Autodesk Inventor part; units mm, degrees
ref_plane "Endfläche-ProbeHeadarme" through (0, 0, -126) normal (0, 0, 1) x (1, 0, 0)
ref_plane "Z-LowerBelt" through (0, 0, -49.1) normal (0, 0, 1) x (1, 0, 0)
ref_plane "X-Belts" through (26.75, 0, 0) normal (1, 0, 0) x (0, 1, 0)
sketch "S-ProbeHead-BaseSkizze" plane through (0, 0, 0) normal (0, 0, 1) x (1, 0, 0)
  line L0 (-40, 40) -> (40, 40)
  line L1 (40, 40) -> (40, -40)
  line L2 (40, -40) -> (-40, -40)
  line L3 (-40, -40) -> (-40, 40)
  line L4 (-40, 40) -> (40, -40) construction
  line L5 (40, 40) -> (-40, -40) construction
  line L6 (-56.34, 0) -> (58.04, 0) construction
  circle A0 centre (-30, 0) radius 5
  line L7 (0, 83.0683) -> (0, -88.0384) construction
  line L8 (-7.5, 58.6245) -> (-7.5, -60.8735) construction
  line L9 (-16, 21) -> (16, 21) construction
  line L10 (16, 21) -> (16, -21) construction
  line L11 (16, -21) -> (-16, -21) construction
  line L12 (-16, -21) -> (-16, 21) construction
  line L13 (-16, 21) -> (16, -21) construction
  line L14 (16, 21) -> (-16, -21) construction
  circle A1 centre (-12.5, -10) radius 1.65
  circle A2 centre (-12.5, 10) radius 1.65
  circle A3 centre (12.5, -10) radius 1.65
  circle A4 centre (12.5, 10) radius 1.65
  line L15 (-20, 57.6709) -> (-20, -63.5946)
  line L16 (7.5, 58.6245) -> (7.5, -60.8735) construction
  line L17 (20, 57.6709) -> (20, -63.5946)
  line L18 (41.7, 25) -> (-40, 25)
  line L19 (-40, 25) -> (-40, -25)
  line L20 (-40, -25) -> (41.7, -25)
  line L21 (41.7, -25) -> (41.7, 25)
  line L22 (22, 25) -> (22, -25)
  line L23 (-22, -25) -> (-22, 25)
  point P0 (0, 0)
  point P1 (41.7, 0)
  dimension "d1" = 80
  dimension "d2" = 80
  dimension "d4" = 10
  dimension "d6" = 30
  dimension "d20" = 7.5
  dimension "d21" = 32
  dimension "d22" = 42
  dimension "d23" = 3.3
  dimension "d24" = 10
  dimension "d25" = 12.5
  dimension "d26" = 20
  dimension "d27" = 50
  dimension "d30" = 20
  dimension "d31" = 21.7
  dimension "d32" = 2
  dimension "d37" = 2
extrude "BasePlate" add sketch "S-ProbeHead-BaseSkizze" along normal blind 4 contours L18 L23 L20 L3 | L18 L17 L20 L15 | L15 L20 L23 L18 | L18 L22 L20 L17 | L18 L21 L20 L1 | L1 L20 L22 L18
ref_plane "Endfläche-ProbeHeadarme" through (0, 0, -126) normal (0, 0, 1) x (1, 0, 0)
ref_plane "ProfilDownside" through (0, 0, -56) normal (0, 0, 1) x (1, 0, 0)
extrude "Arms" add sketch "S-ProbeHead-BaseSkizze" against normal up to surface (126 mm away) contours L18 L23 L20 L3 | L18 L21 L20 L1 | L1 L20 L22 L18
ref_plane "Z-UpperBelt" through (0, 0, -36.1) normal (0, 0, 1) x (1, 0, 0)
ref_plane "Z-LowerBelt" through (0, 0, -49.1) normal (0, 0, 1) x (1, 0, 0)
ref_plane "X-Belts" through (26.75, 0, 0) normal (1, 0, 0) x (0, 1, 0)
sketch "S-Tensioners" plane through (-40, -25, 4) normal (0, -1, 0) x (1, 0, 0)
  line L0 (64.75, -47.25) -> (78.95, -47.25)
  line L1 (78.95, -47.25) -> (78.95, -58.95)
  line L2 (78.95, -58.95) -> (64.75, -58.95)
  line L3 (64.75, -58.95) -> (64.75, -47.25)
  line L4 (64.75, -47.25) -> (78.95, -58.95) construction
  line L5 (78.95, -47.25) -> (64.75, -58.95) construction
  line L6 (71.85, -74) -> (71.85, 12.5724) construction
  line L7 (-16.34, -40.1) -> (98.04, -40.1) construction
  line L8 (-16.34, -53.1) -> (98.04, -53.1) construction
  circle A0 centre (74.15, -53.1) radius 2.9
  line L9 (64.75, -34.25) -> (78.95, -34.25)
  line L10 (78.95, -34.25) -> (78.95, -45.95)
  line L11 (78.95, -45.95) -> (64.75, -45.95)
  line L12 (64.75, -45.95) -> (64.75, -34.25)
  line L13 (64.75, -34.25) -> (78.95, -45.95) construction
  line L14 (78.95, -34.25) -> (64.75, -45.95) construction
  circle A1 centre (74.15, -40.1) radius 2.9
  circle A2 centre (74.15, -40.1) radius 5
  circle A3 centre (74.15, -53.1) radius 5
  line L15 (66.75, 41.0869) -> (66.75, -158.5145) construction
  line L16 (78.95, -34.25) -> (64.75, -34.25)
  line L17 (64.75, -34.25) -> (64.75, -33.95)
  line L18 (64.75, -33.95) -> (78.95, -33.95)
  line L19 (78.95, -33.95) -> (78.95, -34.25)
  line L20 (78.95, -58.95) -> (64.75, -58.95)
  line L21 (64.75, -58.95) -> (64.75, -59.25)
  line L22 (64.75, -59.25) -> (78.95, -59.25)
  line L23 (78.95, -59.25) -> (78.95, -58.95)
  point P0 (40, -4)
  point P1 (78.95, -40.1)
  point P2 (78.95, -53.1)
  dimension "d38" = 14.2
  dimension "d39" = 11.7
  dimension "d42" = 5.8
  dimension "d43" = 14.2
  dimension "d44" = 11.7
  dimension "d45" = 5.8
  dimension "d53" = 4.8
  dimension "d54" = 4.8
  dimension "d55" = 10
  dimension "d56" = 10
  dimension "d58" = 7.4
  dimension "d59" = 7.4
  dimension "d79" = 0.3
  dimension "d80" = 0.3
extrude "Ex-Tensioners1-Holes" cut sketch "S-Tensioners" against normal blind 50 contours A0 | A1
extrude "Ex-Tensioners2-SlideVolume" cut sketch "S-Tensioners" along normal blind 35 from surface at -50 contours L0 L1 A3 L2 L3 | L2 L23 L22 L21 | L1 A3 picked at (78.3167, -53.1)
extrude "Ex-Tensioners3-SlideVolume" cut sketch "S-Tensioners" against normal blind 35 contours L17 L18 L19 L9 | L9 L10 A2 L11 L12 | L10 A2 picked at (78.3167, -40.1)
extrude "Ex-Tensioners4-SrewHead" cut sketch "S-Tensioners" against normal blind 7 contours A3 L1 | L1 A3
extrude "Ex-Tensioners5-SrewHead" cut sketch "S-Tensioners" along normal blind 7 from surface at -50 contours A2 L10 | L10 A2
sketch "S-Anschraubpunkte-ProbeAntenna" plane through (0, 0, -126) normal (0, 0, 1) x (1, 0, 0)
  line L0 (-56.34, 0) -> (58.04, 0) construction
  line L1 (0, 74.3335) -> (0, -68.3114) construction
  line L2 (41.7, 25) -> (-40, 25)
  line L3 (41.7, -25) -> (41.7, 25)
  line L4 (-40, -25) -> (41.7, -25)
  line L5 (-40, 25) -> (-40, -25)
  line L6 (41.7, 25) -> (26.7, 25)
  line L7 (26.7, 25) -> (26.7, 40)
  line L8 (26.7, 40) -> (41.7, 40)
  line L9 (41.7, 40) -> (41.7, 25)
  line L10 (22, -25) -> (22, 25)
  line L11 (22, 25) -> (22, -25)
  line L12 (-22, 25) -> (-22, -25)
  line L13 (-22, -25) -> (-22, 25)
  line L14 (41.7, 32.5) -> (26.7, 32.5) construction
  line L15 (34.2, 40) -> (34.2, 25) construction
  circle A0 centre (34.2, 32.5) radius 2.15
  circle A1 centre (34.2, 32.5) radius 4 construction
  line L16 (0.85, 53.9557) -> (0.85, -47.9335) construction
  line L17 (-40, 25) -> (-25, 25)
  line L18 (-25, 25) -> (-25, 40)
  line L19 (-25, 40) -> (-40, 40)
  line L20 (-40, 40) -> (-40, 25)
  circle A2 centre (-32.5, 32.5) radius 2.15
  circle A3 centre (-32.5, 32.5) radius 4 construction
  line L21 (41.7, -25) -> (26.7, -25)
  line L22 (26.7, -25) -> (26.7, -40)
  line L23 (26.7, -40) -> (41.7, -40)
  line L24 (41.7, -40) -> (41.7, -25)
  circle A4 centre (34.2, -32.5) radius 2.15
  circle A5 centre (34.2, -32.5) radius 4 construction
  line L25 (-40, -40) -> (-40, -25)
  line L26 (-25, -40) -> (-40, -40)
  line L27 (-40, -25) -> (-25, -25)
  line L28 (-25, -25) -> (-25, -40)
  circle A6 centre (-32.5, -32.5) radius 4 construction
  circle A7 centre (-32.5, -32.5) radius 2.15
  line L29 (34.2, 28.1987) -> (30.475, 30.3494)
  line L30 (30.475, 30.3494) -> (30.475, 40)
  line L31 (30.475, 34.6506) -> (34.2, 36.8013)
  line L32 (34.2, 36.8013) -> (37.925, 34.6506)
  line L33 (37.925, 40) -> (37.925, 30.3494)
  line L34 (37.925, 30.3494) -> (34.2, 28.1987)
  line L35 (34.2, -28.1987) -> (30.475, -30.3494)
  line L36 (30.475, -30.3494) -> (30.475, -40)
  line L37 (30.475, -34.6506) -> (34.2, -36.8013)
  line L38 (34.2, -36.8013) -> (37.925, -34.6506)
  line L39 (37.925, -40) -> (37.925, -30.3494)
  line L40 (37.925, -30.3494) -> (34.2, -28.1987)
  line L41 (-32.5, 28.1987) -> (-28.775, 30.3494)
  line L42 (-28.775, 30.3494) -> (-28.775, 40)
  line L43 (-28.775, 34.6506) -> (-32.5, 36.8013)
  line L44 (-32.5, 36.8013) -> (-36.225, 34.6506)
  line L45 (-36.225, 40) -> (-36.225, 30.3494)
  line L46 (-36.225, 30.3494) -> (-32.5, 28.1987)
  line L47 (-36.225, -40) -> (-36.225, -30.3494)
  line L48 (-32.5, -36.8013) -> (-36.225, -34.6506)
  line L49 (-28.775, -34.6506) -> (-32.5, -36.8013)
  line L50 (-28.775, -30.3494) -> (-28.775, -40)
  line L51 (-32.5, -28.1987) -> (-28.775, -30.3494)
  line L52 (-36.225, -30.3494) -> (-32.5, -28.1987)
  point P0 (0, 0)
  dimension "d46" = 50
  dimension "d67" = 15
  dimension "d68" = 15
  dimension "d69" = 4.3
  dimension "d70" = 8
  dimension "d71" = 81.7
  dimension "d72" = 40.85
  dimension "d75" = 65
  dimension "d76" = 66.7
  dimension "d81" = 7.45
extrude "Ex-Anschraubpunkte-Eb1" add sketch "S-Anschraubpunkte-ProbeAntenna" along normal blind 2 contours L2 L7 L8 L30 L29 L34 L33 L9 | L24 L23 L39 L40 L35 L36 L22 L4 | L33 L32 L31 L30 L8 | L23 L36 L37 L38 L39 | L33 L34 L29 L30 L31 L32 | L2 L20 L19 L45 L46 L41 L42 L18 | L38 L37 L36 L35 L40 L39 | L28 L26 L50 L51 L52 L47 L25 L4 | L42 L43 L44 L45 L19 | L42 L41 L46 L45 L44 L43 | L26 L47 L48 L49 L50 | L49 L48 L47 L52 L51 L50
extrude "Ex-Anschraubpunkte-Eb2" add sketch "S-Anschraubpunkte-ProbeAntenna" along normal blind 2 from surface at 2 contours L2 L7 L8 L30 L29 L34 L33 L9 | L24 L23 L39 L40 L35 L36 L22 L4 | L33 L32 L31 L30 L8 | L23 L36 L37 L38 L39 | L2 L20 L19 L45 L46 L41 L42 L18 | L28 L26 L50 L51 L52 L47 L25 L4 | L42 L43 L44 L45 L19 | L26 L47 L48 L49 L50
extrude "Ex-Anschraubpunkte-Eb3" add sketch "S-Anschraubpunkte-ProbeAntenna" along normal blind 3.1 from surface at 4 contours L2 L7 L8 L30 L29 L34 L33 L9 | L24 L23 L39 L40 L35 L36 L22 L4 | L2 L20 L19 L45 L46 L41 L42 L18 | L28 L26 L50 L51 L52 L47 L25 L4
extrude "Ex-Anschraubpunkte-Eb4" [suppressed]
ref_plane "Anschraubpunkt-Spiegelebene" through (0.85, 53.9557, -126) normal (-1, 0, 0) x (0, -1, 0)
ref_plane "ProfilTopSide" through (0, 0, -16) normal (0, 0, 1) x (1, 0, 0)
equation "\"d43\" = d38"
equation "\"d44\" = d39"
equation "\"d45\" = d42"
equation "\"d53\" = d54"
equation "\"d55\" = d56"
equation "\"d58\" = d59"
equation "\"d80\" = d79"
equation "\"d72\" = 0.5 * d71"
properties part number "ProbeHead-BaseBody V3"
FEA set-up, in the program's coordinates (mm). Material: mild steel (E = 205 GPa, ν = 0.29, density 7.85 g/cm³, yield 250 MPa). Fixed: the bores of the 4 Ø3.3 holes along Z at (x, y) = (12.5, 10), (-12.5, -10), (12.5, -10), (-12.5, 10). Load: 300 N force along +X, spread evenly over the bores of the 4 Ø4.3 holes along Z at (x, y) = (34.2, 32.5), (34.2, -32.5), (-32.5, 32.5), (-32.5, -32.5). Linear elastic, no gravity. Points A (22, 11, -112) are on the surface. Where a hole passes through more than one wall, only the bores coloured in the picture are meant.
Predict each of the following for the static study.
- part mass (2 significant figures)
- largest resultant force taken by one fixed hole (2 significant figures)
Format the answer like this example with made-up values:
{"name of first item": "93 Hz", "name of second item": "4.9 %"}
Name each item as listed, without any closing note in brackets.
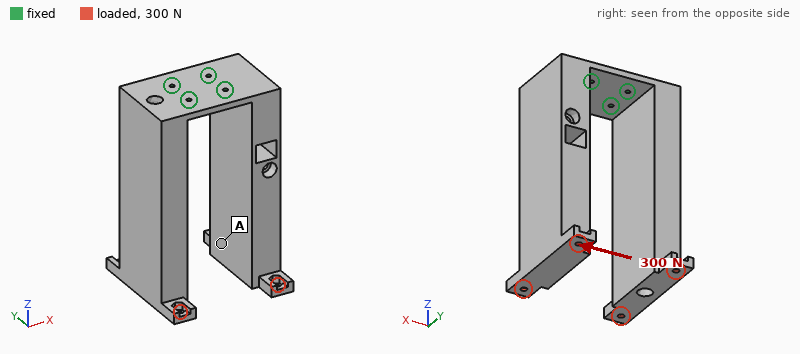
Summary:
{"part mass": "1.8 kg", "largest resultant force taken by one fixed hole": "290 N"}
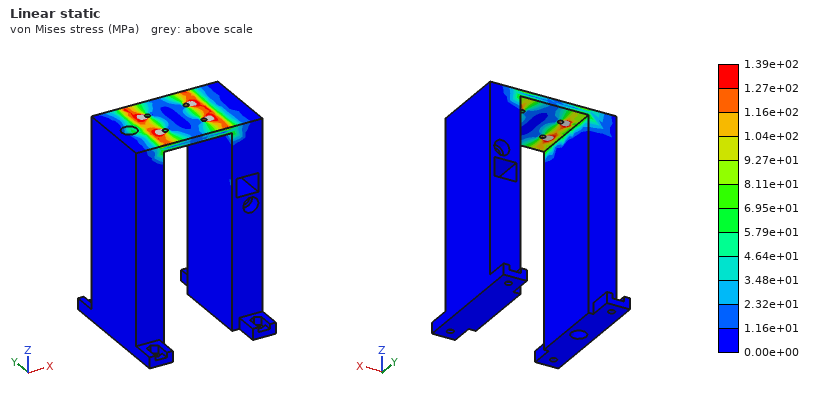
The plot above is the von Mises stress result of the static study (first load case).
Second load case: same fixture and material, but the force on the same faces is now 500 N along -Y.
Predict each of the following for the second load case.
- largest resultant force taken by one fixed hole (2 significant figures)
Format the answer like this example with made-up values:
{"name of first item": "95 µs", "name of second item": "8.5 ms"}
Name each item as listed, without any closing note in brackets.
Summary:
{"largest resultant force taken by one fixed hole": "1.3 kN"}
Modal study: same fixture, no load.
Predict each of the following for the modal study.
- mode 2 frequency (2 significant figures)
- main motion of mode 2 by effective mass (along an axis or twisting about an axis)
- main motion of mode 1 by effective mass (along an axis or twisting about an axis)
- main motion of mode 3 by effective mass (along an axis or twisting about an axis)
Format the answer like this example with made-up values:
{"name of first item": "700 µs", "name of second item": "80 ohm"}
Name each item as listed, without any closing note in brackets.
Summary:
{"mode 2 frequency": "150 Hz", "main motion of mode 2 by effective mass": "along X", "main motion of mode 1 by effective mass": "along X", "main motion of mode 3 by effective mass": "along Y"}
